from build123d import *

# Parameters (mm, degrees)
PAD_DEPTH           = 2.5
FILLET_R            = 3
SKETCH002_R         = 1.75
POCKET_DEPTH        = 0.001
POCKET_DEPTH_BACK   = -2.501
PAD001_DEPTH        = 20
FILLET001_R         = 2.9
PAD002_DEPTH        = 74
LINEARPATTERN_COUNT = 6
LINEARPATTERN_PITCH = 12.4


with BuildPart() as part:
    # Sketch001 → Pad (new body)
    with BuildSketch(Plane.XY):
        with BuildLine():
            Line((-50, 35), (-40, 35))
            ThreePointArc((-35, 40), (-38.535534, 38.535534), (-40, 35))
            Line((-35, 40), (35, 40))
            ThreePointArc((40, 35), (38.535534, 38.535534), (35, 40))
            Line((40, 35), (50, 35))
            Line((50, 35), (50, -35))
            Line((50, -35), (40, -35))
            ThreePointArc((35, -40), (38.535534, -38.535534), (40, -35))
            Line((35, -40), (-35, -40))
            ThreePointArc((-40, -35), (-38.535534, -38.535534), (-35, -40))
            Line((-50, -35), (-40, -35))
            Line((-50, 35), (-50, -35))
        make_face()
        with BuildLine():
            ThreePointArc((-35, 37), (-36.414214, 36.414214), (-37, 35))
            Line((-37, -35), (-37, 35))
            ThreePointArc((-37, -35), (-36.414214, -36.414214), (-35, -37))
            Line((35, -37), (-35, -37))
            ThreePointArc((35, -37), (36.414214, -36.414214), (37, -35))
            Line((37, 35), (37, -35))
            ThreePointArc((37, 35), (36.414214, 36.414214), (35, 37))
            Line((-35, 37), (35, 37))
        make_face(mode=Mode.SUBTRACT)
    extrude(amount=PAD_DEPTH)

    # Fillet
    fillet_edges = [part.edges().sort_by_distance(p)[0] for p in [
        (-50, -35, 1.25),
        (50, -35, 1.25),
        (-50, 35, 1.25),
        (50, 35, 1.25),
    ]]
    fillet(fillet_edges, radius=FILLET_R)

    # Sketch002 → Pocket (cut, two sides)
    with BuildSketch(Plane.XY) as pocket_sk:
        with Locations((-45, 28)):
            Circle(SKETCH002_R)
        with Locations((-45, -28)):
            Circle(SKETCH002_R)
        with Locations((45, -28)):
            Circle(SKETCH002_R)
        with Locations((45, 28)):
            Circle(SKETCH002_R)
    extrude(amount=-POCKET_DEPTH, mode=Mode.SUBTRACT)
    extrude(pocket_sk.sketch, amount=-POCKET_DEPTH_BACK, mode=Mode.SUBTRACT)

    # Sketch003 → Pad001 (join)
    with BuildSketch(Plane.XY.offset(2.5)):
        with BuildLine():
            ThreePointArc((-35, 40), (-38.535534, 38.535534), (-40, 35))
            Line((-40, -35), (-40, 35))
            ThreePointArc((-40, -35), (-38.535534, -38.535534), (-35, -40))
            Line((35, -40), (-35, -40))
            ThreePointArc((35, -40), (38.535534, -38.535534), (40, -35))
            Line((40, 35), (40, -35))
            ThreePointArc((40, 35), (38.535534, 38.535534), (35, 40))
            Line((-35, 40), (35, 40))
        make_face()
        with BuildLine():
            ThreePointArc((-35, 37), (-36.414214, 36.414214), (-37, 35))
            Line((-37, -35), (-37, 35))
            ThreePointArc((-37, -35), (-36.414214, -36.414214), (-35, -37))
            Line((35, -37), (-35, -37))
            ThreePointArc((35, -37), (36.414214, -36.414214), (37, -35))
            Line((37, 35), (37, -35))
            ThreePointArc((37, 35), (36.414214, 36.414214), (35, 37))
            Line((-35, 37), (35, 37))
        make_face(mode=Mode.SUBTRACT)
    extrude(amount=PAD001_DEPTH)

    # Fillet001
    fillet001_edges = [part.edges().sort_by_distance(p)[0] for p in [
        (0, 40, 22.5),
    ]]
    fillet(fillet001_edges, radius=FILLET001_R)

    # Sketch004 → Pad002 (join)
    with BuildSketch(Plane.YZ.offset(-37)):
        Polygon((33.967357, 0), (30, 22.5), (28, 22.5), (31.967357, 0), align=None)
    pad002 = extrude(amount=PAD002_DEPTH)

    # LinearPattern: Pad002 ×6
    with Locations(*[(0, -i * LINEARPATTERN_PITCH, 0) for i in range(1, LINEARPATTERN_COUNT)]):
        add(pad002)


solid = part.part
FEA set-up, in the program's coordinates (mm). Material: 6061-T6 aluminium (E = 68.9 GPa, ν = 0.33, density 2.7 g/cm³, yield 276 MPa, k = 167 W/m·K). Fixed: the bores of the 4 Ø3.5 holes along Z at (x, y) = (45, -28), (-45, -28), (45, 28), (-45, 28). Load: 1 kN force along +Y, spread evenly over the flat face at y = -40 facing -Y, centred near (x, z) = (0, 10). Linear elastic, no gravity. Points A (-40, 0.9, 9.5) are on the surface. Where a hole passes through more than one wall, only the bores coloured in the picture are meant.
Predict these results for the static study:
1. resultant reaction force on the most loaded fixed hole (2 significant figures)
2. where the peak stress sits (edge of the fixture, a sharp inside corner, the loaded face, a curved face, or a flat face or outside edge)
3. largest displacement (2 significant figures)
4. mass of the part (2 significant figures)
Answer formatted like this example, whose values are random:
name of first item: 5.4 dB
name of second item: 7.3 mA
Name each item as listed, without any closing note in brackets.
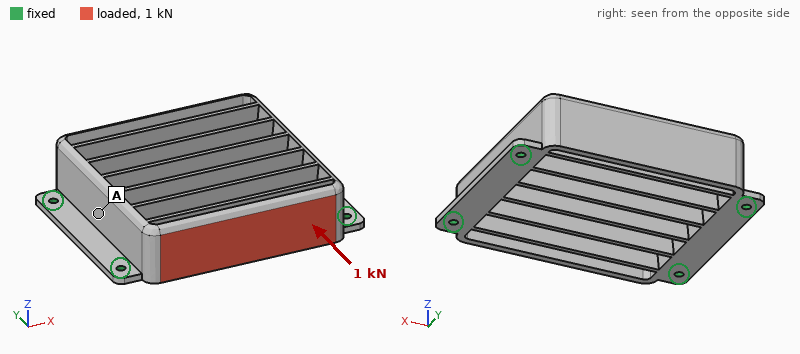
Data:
resultant reaction force on the most loaded fixed hole: 450 N
where the peak stress sits: a curved face
largest displacement: 0.46 mm
mass of the part: 120 g
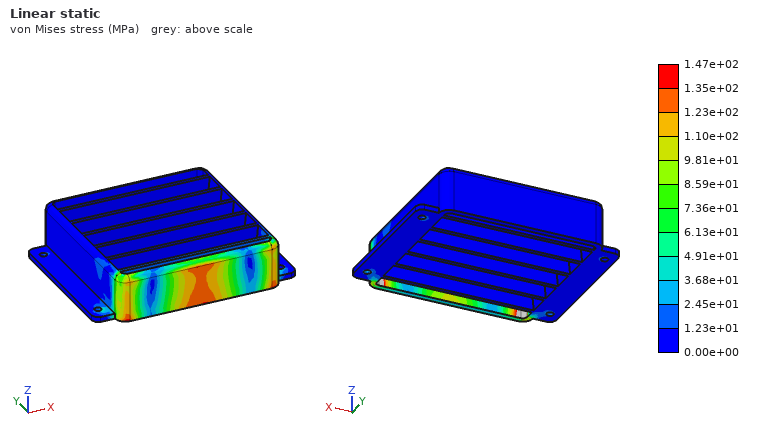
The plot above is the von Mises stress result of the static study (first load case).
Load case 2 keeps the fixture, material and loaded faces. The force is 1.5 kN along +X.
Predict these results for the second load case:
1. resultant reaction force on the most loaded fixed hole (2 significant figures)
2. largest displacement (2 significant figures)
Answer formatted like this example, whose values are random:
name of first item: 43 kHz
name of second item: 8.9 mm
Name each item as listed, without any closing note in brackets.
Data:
resultant reaction force on the most loaded fixed hole: 850 N
largest displacement: 63 µm
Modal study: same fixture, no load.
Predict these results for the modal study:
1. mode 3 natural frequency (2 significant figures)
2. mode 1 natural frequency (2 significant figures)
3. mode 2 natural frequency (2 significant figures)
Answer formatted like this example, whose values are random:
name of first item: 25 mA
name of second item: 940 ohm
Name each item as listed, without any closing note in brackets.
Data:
mode 3 natural frequency: 1800 Hz
mode 1 natural frequency: 1800 Hz
mode 2 natural frequency: 1800 Hz
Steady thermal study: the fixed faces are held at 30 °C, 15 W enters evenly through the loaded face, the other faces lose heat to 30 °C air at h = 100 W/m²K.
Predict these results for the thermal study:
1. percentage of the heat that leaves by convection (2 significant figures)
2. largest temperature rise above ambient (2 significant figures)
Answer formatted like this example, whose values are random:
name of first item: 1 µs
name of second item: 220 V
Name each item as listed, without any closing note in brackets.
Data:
percentage of the heat that leaves by convection: 53 %
largest temperature rise above ambient: 19 K
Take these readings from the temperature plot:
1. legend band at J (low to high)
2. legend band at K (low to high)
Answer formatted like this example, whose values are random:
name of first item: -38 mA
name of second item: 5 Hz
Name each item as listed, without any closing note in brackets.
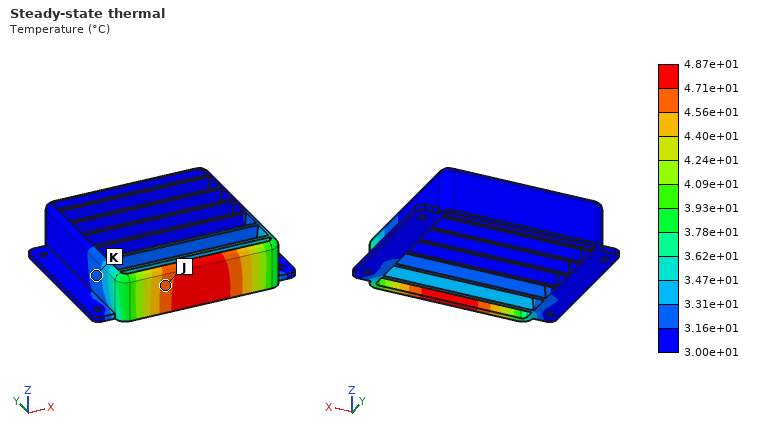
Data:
legend band at J: 4.56e+01 to 4.71e+01 °C
legend band at K: 3.16e+01 to 3.31e+01 °C
